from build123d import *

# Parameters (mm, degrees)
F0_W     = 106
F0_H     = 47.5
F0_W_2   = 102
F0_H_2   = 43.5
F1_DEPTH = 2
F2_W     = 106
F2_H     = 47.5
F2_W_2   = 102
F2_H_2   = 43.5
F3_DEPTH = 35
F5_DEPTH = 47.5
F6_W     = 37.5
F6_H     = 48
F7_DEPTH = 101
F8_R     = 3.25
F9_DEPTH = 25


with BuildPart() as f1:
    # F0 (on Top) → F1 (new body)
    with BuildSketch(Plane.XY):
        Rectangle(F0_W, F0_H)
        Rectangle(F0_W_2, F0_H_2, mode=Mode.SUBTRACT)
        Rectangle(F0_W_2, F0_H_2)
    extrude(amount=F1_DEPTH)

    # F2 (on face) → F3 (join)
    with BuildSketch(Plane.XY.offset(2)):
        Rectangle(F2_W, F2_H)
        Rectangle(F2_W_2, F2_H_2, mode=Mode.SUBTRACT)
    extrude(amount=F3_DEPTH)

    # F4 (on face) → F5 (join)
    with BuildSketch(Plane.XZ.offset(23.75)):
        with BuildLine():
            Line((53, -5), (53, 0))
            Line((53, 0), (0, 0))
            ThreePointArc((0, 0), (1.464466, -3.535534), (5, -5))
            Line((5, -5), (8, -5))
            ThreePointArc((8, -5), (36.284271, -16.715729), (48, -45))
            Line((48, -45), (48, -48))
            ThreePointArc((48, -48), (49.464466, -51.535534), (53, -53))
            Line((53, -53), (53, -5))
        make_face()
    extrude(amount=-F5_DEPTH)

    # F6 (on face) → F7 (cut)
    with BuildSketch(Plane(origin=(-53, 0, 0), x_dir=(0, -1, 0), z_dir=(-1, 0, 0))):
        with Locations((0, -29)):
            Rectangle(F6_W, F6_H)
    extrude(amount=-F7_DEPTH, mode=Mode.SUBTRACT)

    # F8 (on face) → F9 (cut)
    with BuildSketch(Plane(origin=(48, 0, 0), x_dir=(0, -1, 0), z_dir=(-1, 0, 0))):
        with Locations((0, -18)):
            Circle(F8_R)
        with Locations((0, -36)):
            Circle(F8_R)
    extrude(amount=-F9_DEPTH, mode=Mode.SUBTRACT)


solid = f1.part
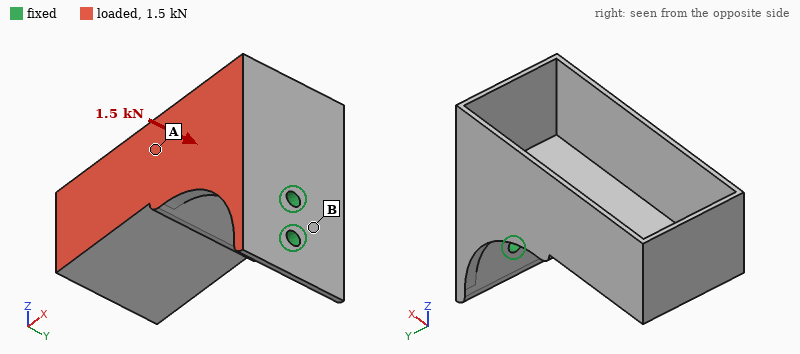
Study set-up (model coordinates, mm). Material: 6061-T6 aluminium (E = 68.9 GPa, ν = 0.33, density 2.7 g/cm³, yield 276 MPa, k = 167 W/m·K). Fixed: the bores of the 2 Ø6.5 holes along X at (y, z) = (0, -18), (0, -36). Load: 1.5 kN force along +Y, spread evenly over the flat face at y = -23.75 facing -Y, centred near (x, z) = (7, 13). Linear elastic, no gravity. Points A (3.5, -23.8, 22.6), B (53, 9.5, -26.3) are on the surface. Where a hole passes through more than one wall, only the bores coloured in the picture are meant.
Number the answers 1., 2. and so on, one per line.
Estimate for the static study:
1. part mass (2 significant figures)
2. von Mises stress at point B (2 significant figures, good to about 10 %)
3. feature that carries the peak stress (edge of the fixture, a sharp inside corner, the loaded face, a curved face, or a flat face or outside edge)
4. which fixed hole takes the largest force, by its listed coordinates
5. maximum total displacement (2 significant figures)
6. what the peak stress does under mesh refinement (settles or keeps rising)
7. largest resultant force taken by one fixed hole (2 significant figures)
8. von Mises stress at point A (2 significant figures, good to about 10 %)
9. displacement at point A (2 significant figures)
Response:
1. 160 g
2. 94 MPa
3. edge of the fixture
4. (0, -18)
5. 1.4 mm
6. keeps rising
7. 3.3 kN
8. 35 MPa
9. 0.88 mm
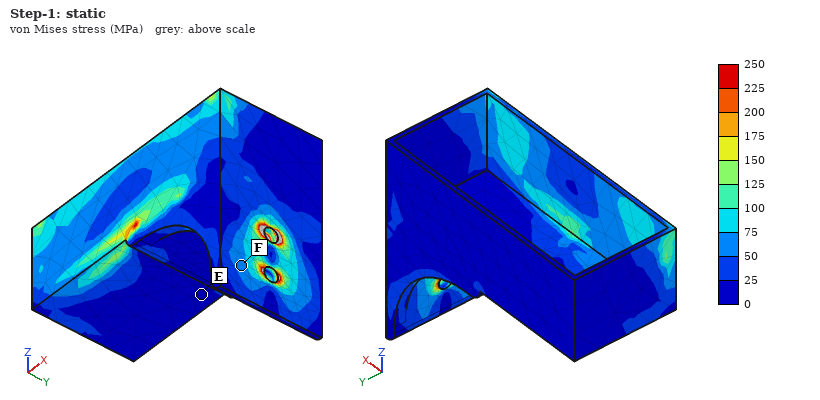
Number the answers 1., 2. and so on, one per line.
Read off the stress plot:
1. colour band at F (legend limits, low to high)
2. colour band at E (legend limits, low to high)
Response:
1. 50 to 75 MPa
2. 0 to 25 MPa
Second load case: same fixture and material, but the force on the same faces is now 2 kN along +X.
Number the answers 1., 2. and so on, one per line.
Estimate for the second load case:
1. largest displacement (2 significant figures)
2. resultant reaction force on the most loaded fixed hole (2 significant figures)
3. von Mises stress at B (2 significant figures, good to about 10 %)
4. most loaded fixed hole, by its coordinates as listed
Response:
1. 1.4 mm
2. 3.7 kN
3. 83 MPa
4. (0, -18)
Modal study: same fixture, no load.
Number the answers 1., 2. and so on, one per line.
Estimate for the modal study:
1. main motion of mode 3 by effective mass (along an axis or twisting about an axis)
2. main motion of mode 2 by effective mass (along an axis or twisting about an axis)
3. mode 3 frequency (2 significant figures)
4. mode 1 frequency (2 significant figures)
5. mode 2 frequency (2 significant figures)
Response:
1. twisting about X
2. along Y
3. 1200 Hz
4. 660 Hz
5. 690 Hz
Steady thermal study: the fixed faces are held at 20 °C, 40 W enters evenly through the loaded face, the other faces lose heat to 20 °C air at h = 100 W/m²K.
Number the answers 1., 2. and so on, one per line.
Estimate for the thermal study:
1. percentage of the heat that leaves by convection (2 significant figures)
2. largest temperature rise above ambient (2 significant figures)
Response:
1. 65 %
2. 23 K
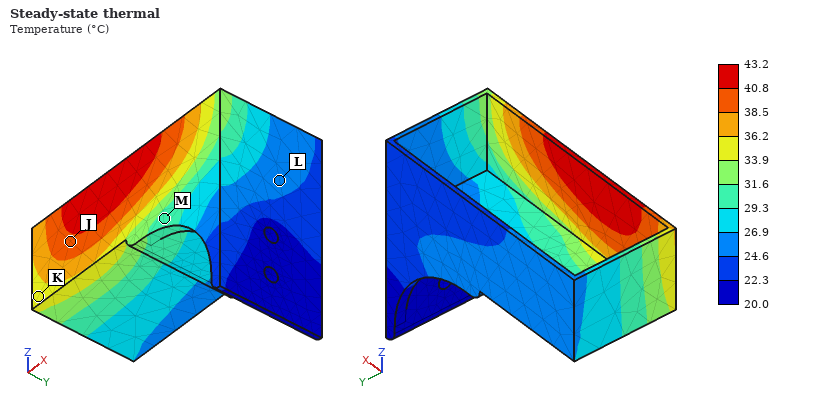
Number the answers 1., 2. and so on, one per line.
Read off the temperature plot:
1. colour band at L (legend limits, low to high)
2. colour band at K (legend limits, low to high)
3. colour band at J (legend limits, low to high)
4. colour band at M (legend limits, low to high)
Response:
1. 24.6 to 26.9 °C
2. 33.9 to 36.2 °C
3. 38.5 to 40.8 °C
4. 29.3 to 31.6 °C
